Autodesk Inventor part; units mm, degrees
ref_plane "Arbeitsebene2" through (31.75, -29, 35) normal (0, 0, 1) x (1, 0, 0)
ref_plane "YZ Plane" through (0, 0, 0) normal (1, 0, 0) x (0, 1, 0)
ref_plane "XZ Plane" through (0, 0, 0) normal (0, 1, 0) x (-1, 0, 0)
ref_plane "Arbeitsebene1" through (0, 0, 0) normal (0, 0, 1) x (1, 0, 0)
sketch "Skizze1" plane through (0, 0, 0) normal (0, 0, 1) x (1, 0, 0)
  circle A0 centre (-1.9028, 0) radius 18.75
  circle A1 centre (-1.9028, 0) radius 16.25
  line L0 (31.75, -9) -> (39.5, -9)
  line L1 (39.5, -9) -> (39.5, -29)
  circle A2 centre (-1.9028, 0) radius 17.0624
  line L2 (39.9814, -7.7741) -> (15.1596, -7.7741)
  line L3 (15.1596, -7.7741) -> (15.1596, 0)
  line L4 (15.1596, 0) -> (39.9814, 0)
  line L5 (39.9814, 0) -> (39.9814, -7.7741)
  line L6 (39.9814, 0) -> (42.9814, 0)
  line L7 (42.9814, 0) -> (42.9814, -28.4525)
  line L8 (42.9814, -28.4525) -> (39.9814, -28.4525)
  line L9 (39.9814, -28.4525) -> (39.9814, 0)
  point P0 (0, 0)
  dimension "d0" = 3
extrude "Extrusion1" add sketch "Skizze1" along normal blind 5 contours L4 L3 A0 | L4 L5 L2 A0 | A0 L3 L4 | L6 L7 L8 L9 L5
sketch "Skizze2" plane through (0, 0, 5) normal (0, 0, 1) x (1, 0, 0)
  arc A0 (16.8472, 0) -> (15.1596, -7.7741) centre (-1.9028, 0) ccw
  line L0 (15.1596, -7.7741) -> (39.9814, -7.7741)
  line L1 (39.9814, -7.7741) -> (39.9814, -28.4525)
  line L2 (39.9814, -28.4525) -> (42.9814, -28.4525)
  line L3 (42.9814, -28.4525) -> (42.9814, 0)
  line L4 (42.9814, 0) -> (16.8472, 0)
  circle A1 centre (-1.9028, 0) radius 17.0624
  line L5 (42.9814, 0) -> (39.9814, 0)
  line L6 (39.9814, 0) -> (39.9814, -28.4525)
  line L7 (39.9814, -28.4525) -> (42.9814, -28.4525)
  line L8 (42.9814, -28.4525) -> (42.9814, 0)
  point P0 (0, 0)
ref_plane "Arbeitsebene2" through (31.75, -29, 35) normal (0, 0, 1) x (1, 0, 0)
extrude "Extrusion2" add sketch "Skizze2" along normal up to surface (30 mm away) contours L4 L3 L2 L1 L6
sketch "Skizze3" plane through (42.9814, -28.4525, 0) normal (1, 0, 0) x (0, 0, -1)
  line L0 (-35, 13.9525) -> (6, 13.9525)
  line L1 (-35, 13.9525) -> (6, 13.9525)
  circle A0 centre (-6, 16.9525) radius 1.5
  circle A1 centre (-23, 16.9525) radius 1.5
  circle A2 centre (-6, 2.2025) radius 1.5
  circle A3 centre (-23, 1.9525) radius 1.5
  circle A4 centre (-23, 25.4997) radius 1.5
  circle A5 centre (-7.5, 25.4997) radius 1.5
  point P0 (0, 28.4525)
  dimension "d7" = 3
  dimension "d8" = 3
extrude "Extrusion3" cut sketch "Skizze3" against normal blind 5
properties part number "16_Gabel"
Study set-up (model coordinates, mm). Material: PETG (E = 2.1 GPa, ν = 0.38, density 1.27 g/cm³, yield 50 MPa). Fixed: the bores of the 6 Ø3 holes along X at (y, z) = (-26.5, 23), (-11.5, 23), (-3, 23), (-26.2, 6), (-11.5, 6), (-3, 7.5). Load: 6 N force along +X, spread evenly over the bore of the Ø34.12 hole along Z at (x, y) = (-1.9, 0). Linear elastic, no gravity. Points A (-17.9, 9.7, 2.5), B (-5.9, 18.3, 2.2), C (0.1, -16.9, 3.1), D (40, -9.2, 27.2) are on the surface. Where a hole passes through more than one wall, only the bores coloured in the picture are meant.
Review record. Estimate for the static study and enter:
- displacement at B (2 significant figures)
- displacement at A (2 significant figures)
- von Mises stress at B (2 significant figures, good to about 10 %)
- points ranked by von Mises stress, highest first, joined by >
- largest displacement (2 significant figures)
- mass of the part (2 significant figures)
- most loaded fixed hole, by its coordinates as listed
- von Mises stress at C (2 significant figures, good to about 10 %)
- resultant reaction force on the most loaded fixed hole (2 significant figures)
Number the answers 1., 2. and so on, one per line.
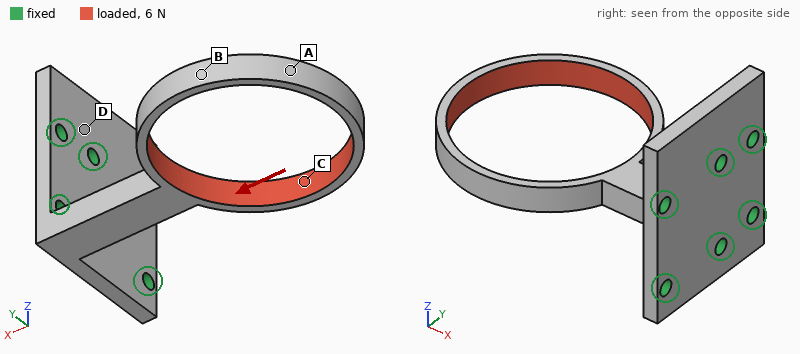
1. 0.91 mm
2. 0.92 mm
3. 2.7 MPa
4. C > B > A > D
5. 0.92 mm
6. 6.0 g
7. (-3, 7.5)
8. 4.2 MPa
9. 6.9 N
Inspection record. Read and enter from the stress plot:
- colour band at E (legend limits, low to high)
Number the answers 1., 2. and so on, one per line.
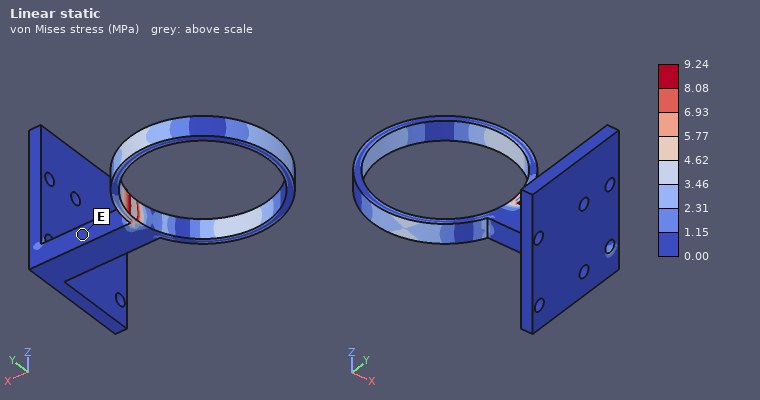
1. 0.00 to 1.15 MPa
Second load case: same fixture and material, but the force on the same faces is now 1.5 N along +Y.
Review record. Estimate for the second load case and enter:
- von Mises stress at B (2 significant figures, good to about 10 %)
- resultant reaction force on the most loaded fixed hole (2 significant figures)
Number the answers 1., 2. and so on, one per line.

1. 1.4 MPa
2. 6.8 N
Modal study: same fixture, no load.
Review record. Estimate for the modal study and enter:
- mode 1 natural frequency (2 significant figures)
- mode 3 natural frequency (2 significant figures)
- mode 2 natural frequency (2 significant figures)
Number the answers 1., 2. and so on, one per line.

1. 190 Hz
2. 570 Hz
3. 190 Hz
